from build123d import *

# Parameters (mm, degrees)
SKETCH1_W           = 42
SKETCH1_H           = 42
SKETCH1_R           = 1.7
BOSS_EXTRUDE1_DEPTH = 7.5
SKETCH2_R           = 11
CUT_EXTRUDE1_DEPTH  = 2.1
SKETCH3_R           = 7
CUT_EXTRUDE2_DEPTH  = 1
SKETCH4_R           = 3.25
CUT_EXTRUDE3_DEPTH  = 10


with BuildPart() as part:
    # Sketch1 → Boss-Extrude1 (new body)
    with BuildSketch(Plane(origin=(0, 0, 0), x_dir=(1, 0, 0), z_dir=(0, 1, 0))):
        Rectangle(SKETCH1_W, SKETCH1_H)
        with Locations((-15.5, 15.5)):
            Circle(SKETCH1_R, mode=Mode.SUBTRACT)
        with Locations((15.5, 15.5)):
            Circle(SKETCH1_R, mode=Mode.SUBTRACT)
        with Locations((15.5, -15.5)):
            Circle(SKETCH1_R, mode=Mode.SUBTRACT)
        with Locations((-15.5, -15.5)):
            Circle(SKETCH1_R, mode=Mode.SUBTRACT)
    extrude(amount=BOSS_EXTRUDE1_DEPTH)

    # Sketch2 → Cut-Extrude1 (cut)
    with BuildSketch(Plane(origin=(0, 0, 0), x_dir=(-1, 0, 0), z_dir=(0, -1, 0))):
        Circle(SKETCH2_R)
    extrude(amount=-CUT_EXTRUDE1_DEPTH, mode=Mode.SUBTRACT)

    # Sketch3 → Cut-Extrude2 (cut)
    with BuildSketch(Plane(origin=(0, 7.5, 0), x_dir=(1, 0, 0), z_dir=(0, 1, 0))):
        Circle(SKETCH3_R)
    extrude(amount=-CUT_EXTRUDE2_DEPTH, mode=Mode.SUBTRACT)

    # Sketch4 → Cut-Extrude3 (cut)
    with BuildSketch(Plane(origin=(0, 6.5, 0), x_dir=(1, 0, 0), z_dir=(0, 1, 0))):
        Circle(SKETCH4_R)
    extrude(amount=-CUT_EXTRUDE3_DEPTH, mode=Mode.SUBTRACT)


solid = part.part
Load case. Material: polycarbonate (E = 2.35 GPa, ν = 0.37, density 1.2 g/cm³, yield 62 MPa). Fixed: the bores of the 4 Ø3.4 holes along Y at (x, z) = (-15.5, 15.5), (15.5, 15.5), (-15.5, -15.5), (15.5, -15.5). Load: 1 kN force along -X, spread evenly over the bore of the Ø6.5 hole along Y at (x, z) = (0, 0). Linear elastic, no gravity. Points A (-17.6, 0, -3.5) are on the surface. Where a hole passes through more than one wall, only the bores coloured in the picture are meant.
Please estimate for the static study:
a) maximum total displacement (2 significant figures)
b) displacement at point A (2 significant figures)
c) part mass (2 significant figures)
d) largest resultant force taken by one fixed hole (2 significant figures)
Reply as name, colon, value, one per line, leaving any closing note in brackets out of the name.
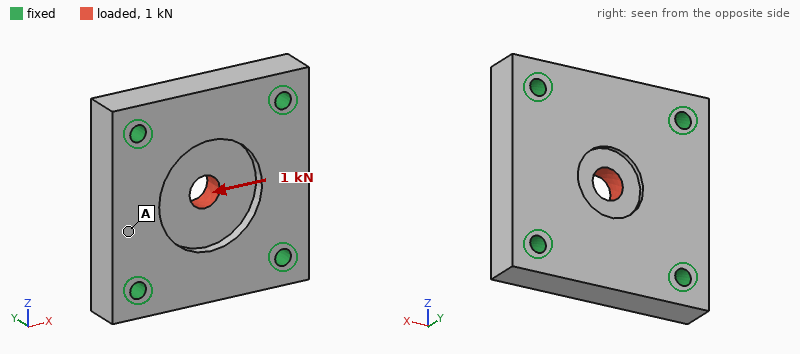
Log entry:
maximum total displacement: 58 µm
displacement at point A: 24 µm
part mass: 14 g
largest resultant force taken by one fixed hole: 280 N
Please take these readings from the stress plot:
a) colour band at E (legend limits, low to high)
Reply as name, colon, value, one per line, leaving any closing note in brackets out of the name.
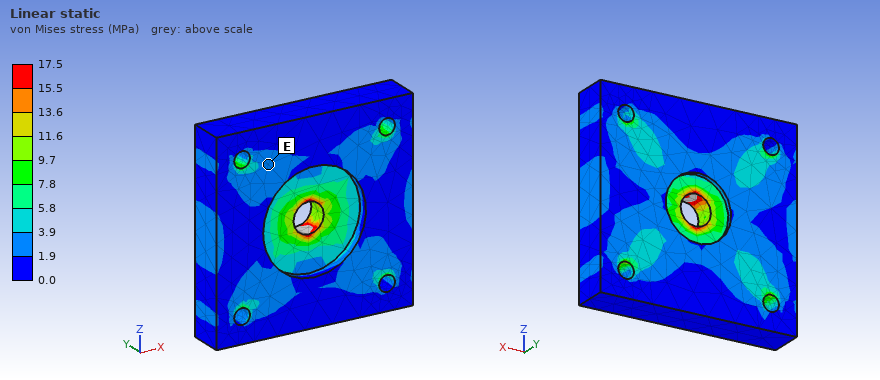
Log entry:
colour band at E: 1.9 to 3.9 MPa
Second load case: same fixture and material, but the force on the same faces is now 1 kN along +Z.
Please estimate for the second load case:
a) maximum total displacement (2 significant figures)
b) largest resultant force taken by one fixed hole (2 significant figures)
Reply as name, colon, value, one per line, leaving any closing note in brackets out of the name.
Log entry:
maximum total displacement: 58 µm
largest resultant force taken by one fixed hole: 280 N
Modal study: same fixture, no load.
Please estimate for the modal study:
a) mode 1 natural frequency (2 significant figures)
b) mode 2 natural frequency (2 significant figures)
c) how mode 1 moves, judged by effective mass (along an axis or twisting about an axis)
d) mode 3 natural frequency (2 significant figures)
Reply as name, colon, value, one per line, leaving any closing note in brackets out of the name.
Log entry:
mode 1 natural frequency: 6200 Hz
mode 2 natural frequency: 8800 Hz
how mode 1 moves, judged by effective mass: along Y
mode 3 natural frequency: 8800 Hz
